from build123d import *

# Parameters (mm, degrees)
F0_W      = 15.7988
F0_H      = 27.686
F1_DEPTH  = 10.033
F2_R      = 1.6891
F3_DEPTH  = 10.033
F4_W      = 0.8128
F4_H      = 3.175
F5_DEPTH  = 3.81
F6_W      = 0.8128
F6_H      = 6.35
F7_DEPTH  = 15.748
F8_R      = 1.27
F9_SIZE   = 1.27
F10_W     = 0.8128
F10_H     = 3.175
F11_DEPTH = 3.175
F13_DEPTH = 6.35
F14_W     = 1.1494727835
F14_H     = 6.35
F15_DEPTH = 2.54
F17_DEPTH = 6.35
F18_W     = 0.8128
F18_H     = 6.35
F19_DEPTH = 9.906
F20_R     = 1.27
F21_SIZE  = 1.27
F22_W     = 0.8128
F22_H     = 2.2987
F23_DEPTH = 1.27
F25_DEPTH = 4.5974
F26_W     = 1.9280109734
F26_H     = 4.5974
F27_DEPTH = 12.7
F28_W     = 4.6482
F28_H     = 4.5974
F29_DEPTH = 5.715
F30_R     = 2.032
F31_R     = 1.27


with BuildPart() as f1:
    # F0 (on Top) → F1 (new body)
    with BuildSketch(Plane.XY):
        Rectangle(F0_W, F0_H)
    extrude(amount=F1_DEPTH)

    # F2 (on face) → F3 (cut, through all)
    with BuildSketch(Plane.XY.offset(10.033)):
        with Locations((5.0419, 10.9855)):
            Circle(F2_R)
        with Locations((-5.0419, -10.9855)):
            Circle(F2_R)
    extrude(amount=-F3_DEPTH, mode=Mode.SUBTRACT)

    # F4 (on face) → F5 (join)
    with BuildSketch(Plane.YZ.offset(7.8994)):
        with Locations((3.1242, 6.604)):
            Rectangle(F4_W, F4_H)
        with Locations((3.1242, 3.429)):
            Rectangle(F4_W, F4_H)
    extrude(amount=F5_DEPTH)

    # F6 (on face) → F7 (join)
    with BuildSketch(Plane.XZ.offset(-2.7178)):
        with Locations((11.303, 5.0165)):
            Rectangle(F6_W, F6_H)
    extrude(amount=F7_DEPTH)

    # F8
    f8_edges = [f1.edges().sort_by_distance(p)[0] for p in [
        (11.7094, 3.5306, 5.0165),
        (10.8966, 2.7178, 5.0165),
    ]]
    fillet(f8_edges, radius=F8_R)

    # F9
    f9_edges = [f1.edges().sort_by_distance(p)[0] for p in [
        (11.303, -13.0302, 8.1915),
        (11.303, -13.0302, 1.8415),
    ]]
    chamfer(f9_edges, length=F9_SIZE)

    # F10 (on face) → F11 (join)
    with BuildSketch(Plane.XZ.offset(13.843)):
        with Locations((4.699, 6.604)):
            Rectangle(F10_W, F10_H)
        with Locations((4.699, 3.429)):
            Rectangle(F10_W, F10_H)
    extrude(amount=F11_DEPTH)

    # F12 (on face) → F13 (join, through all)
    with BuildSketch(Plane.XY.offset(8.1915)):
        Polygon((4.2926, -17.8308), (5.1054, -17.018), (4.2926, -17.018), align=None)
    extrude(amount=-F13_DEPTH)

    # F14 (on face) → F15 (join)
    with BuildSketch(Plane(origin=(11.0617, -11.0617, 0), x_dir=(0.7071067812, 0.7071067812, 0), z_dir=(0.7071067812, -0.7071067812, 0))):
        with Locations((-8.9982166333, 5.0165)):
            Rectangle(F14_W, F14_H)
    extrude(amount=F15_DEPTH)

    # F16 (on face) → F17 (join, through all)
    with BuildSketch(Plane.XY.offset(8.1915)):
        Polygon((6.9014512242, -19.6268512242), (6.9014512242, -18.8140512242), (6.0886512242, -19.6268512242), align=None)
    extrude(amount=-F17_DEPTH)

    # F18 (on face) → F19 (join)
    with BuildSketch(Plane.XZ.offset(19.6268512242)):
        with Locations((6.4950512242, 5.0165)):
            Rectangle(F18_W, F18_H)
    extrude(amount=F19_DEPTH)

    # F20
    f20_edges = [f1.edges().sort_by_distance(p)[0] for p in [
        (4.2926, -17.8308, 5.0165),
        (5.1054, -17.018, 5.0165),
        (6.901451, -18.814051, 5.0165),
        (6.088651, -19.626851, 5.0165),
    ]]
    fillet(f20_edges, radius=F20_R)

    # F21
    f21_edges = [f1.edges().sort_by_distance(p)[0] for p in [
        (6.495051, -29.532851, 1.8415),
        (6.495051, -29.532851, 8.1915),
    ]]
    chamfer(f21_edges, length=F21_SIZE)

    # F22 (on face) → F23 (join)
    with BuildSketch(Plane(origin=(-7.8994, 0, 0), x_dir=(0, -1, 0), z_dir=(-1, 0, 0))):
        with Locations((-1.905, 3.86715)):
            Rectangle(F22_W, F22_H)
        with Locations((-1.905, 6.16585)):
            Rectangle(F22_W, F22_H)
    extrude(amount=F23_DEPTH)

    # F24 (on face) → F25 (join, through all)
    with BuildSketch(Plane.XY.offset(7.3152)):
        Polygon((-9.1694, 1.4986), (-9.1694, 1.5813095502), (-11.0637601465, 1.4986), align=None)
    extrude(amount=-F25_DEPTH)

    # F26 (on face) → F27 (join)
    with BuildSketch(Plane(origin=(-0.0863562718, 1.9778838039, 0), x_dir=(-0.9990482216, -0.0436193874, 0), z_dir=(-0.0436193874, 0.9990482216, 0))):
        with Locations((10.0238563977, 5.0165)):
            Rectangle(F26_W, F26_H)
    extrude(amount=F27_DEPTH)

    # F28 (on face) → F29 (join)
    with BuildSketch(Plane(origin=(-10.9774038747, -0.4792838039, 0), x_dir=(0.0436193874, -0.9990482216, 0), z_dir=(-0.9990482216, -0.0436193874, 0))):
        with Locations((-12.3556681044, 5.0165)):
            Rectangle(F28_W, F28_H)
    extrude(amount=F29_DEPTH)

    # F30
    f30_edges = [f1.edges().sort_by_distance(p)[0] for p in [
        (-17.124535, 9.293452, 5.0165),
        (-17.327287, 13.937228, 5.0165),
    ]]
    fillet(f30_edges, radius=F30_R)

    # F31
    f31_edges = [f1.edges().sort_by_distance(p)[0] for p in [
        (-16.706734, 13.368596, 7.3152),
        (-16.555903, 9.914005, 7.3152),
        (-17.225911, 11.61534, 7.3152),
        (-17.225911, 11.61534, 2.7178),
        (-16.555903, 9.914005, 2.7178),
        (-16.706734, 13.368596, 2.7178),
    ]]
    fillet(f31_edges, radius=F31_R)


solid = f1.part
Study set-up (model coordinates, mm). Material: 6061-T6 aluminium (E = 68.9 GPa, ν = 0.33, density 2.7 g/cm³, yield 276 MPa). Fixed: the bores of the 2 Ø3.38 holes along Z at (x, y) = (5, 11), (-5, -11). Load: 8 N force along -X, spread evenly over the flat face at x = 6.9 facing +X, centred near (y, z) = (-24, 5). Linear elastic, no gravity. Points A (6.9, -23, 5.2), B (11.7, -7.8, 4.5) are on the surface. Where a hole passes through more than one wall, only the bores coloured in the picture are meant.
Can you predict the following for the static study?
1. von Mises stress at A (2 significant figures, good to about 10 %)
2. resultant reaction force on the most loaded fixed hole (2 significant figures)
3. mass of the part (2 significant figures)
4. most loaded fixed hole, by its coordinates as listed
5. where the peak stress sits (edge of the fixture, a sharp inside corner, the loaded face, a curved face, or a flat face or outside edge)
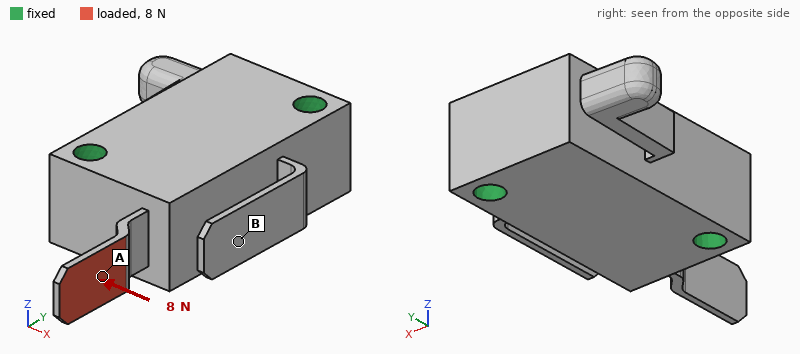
21 MPa
12 N
12 g
(-5, -11)
a flat face or outside edge
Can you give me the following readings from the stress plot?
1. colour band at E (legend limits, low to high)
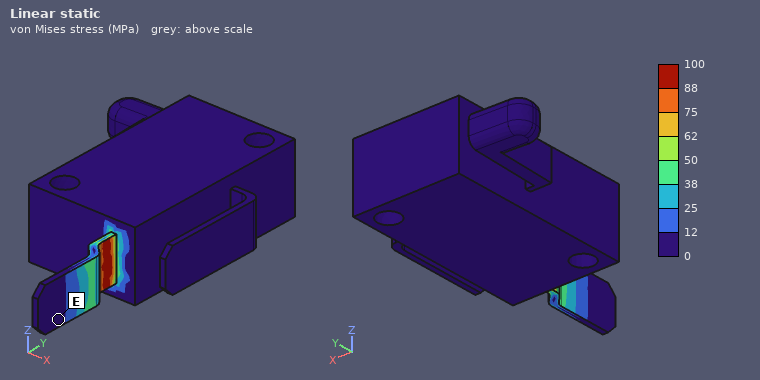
0 to 12 MPa
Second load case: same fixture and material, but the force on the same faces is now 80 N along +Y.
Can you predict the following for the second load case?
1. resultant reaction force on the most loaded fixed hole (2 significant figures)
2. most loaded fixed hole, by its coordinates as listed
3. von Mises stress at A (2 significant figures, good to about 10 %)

51 N
(5, 11)
37 MPa
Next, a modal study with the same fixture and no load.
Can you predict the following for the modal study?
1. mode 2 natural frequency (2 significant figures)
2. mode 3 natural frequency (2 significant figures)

2200 Hz
2900 Hz
